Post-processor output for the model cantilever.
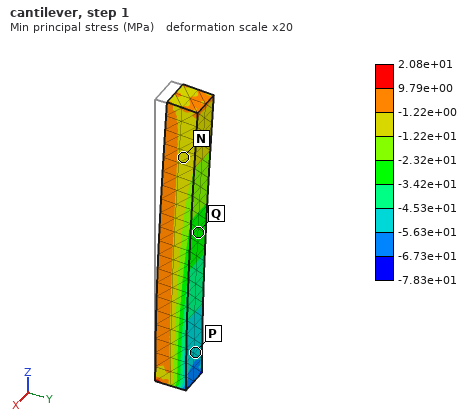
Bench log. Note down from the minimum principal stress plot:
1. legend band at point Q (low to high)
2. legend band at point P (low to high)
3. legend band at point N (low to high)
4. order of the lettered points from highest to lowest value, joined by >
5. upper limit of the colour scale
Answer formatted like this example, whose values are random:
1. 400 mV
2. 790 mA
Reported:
1. -3.42e+01 to -2.32e+01 MPa
2. -5.63e+01 to -4.53e+01 MPa
3. -1.22e+01 to -1.22e+00 MPa
4. N > Q > P
5. 2.08e+01 MPa
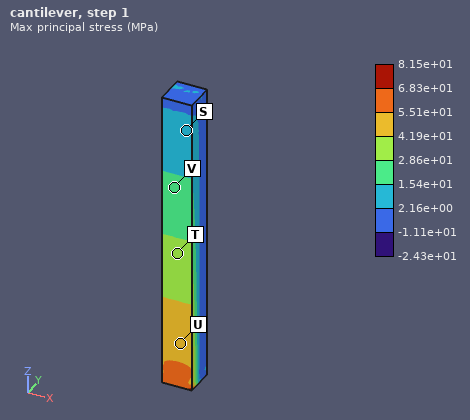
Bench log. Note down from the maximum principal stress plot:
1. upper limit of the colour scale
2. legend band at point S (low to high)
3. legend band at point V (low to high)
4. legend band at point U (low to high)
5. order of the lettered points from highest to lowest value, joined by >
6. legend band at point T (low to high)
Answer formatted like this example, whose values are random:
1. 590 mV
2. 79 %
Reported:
1. 8.15e+01 MPa
2. 2.16e+00 to 1.54e+01 MPa
3. 1.54e+01 to 2.86e+01 MPa
4. 4.19e+01 to 5.51e+01 MPa
5. U > T > V > S
6. 2.86e+01 to 4.19e+01 MPa
